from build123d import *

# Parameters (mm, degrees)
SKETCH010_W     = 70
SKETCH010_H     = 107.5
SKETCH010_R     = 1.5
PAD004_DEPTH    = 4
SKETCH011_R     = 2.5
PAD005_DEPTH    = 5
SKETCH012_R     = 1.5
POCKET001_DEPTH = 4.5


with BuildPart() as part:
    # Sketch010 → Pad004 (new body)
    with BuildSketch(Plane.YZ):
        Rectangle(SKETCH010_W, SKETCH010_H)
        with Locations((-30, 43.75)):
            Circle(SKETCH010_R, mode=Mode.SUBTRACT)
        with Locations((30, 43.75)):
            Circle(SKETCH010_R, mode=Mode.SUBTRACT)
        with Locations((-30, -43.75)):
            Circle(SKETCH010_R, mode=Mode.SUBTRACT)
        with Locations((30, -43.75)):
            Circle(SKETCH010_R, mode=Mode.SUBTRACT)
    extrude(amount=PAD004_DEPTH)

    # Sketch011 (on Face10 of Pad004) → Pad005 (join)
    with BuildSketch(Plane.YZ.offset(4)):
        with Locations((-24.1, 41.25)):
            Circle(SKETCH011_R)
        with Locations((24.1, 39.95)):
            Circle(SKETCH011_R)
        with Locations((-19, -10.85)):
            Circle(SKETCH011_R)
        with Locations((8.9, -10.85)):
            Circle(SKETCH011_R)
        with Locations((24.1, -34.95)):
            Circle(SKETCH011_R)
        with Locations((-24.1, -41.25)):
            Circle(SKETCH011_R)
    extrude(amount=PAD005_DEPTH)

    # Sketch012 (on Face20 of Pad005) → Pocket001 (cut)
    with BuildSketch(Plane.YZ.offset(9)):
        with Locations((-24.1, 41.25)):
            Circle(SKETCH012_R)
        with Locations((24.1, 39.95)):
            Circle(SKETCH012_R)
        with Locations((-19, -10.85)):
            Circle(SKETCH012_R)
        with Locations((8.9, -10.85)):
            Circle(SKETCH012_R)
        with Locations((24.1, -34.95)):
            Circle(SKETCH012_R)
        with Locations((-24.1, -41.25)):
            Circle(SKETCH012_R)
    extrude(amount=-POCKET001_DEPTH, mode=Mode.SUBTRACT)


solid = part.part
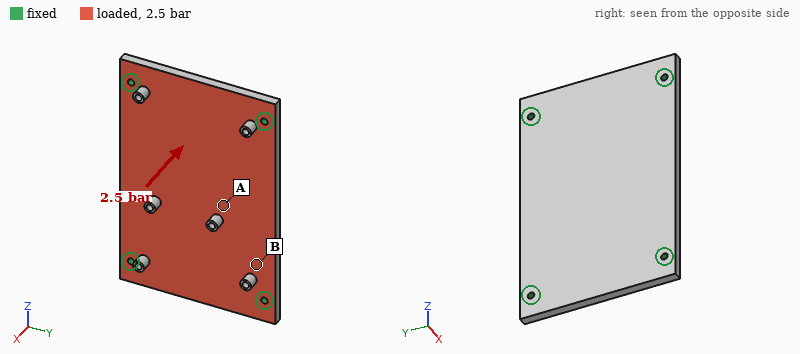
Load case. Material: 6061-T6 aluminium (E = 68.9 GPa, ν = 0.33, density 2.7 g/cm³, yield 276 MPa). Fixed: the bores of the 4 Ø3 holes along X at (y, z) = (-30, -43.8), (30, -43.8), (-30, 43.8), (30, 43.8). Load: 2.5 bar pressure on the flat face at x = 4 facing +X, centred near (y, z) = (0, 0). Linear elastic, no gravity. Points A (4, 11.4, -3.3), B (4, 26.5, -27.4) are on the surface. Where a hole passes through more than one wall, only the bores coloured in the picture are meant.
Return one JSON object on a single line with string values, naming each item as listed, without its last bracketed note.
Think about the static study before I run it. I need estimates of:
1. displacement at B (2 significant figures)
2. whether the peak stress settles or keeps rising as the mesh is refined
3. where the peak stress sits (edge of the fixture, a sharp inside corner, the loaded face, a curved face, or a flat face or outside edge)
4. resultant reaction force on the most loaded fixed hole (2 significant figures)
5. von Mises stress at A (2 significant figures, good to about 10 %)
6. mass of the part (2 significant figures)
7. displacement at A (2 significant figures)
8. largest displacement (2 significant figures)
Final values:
{"displacement at B": "0.071 mm", "whether the peak stress settles or keeps rising as the mesh is refined": "keeps rising", "where the peak stress sits": "edge of the fixture", "resultant reaction force on the most loaded fixed hole": "460 N", "von Mises stress at A": "32 MPa", "mass of the part": "82 g", "displacement at A": "0.17 mm", "largest displacement": "0.17 mm"}
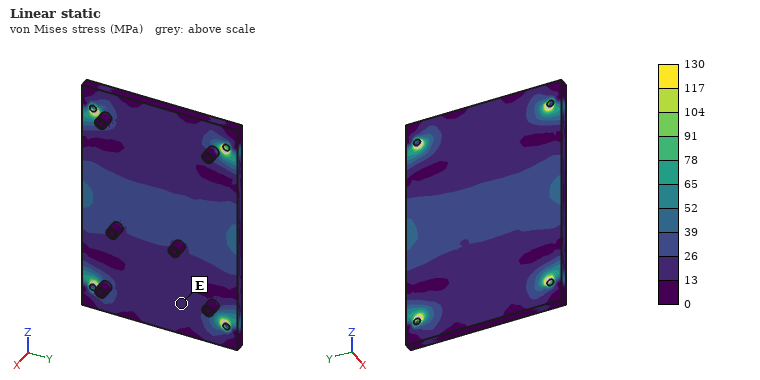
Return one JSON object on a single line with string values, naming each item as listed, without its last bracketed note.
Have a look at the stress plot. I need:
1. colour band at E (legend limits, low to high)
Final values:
{"colour band at E": "13 to 26 MPa"}
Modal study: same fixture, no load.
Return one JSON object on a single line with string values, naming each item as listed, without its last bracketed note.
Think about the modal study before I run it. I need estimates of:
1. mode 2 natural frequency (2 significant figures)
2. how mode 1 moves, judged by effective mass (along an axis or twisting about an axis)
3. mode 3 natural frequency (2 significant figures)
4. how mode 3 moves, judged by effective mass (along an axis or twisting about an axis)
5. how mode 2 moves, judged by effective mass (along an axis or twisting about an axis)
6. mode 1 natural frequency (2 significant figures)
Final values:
{"mode 2 natural frequency": "3400 Hz", "how mode 1 moves, judged by effective mass": "along X", "mode 3 natural frequency": "4900 Hz", "how mode 3 moves, judged by effective mass": "twisting about Y", "how mode 2 moves, judged by effective mass": "twisting about Z", "mode 1 natural frequency": "2100 Hz"}
